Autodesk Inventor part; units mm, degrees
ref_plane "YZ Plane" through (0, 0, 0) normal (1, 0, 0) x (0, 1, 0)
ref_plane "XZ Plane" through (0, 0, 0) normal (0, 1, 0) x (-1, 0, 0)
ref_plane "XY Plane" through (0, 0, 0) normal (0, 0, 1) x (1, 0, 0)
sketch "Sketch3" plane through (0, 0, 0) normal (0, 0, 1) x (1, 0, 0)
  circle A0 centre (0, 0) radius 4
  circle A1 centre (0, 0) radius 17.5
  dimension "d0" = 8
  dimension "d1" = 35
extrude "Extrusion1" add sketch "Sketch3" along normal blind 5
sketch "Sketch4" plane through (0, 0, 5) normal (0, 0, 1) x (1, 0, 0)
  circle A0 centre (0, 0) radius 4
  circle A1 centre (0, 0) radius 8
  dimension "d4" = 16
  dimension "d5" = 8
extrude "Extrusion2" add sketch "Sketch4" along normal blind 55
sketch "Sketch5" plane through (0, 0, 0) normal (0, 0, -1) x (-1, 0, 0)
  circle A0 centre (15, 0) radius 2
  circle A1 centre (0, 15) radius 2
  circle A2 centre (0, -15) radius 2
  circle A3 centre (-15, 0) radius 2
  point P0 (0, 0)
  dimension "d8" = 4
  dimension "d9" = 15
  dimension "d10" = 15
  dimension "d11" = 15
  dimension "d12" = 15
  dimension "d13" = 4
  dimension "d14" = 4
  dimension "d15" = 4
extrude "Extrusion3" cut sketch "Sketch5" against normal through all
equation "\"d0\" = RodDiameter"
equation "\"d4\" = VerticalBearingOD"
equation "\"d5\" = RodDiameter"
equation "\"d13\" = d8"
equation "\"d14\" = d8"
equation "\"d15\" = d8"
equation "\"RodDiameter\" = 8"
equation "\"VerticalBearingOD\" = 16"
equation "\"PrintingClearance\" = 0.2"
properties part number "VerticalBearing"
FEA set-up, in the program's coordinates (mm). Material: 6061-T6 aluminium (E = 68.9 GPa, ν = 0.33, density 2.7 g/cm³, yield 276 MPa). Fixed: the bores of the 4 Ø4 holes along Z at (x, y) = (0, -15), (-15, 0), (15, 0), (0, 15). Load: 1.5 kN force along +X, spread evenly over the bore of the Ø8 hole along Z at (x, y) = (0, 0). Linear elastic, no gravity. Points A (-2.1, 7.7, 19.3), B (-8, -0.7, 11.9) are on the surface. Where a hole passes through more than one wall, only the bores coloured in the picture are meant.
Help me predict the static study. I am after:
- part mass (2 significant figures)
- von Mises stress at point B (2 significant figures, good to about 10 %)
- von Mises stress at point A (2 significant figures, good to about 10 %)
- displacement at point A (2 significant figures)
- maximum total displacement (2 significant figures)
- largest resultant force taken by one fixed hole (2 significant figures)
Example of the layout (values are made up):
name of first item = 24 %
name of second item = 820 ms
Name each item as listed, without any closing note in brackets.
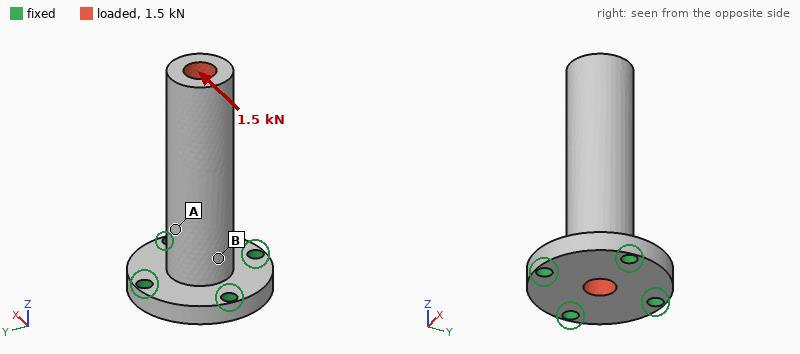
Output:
part mass = 34 g
von Mises stress at point B = 74 MPa
von Mises stress at point A = 23 MPa
displacement at point A = 0.052 mm
maximum total displacement = 0.26 mm
largest resultant force taken by one fixed hole = 1.7 kN
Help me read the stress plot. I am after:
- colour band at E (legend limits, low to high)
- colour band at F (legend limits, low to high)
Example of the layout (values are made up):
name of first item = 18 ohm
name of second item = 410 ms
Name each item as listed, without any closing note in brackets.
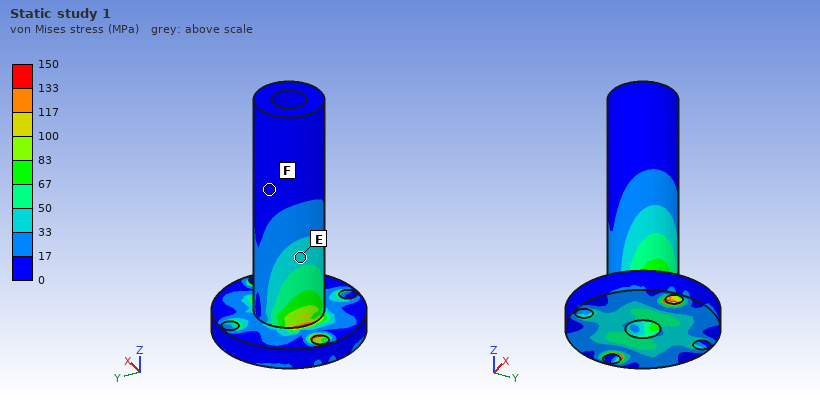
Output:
colour band at E = 33 to 50 MPa
colour band at F = 0 to 17 MPa
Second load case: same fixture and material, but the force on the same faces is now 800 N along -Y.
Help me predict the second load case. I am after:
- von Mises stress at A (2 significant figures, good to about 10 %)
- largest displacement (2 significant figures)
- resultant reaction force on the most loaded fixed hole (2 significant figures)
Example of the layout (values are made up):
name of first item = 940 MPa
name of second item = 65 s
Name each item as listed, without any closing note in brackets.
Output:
von Mises stress at A = 28 MPa
largest displacement = 0.14 mm
resultant reaction force on the most loaded fixed hole = 900 N
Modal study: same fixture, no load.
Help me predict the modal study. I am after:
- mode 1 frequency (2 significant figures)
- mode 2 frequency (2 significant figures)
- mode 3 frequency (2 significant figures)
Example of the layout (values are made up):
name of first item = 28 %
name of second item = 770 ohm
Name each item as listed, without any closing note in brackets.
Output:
mode 1 frequency = 3000 Hz
mode 2 frequency = 3000 Hz
mode 3 frequency = 13 kHz
